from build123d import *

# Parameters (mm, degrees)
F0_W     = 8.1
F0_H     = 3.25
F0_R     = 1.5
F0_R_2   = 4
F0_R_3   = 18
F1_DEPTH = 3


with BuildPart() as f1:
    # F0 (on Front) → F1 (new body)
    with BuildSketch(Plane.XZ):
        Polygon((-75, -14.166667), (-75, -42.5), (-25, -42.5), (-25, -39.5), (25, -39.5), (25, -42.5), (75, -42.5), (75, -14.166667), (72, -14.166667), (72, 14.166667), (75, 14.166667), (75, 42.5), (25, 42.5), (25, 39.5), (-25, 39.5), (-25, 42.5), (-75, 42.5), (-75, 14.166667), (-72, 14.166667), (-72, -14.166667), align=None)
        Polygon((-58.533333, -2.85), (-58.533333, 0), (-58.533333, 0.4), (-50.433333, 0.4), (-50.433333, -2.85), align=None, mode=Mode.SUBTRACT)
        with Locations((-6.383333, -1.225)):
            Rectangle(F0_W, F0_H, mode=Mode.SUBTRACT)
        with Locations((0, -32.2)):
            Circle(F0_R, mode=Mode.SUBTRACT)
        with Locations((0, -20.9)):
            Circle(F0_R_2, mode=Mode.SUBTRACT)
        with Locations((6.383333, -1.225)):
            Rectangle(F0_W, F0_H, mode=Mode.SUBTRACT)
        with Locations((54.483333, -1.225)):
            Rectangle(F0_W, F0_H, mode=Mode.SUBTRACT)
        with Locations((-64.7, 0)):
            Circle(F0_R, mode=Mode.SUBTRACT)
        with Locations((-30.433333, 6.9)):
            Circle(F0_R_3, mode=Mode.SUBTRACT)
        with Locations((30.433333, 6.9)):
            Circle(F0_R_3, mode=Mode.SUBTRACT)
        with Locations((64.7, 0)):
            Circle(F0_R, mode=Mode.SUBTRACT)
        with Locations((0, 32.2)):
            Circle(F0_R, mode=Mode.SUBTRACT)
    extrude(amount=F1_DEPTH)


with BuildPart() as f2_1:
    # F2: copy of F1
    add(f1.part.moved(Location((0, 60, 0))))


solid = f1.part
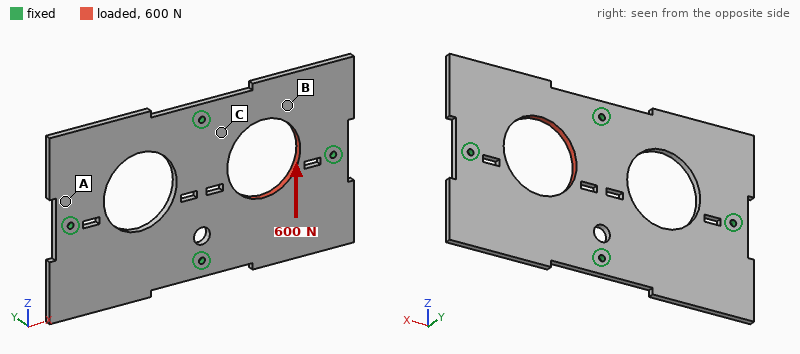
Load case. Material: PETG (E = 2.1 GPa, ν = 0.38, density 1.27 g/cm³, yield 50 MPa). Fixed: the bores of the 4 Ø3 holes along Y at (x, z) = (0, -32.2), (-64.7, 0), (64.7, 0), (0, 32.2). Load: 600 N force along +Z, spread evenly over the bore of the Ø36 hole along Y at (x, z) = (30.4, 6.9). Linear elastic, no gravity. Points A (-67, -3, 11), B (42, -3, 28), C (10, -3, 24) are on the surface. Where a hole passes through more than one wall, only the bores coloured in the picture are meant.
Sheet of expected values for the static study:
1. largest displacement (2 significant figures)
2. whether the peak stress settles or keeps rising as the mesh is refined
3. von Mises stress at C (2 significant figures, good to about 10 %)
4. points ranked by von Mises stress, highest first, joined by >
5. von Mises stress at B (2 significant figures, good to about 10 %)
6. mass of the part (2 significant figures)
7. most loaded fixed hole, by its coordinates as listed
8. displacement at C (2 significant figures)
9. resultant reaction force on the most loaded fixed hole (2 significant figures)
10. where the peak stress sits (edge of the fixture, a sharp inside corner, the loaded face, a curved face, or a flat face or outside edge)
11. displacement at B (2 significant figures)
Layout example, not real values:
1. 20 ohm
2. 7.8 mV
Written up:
1. 0.11 mm
2. keeps rising
3. 3.2 MPa
4. C > B > A
5. 2.2 MPa
6. 38 g
7. (64.7, 0)
8. 0.050 mm
9. 270 N
10. edge of the fixture
11. 0.094 mm
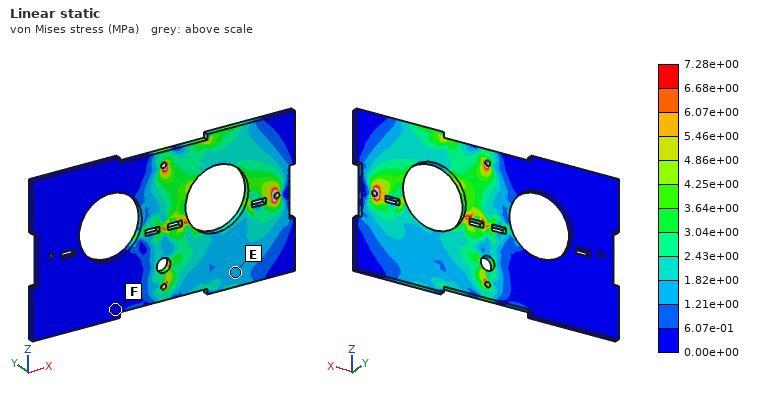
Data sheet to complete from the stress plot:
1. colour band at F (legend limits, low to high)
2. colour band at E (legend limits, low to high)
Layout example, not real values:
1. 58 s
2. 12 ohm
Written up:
1. 0.00e+00 to 6.07e-01 MPa
2. 1.21e+00 to 1.82e+00 MPa
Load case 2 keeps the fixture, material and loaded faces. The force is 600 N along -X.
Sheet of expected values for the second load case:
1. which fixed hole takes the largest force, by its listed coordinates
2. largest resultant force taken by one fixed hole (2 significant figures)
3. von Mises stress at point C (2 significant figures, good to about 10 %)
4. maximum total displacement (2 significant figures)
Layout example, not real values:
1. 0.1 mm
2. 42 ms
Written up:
1. (0, 32.2)
2. 240 N
3. 2.5 MPa
4. 82 µm
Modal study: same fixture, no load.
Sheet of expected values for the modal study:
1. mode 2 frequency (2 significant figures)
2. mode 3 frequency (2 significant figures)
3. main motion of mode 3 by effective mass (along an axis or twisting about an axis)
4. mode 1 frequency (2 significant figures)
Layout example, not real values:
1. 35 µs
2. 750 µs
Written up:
1. 350 Hz
2. 380 Hz
3. twisting about Z
4. 350 Hz
